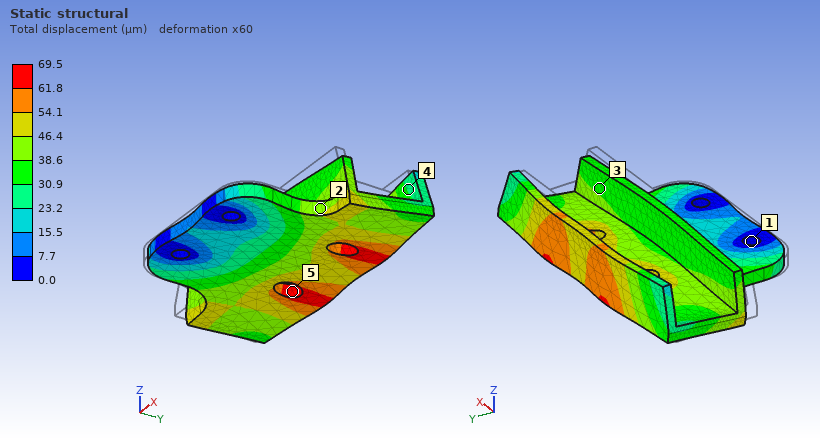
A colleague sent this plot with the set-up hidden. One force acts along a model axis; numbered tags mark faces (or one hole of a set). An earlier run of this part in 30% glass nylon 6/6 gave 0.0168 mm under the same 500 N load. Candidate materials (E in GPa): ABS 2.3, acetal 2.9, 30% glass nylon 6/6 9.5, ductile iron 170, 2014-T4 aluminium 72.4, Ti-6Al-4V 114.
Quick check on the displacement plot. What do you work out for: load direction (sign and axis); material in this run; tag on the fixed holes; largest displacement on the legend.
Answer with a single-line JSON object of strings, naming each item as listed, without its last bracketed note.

{"load direction": "+Y", "material in this run": "ABS", "tag on the fixed holes": "1", "largest displacement on the legend": "69.5 µm"}
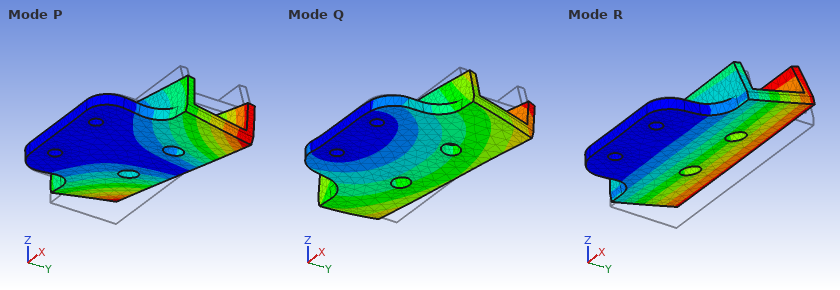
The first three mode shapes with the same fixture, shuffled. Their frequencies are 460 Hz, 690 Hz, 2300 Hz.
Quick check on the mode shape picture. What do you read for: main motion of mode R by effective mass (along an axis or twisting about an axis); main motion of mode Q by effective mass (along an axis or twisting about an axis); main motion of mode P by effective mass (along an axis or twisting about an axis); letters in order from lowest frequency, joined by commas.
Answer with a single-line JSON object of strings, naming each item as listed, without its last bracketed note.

{"main motion of mode R by effective mass": "along Z", "main motion of mode Q by effective mass": "along X", "main motion of mode P by effective mass": "twisting about Y", "letters in order from lowest frequency, joined by commas": "R, P, Q"}
